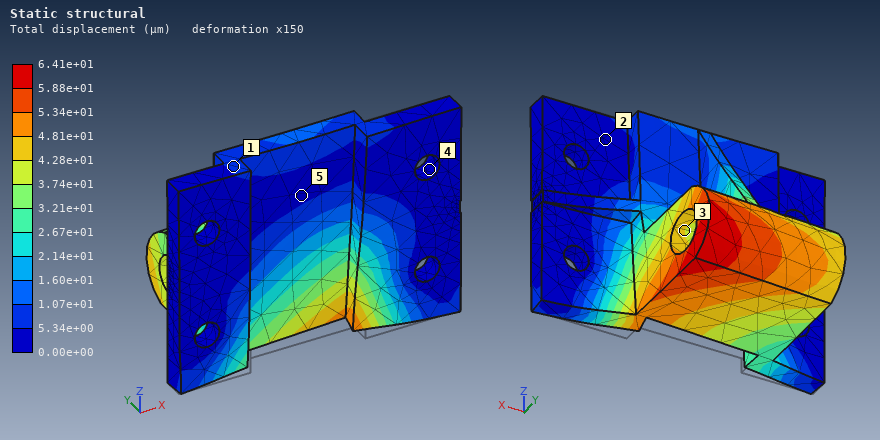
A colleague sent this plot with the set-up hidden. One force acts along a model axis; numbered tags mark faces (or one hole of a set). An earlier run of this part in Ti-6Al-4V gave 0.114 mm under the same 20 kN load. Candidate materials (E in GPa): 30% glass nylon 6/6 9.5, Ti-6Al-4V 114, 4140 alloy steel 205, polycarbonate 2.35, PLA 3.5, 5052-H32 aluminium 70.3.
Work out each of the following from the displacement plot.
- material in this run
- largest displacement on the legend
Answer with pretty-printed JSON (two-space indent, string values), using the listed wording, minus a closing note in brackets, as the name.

{
  "material in this run": "4140 alloy steel",
  "largest displacement on the legend": "6.41e+01 µm"
}
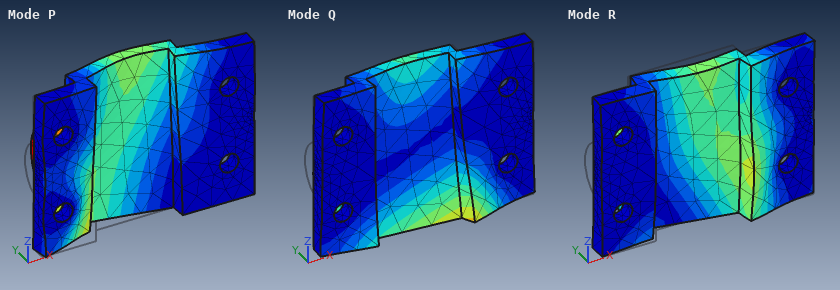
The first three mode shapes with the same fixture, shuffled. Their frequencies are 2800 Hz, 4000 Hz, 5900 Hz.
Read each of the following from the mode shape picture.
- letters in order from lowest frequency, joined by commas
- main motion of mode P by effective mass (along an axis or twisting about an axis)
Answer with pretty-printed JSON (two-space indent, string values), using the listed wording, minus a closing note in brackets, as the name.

{
  "letters in order from lowest frequency, joined by commas": "Q, R, P",
  "main motion of mode P by effective mass": "along Y"
}
